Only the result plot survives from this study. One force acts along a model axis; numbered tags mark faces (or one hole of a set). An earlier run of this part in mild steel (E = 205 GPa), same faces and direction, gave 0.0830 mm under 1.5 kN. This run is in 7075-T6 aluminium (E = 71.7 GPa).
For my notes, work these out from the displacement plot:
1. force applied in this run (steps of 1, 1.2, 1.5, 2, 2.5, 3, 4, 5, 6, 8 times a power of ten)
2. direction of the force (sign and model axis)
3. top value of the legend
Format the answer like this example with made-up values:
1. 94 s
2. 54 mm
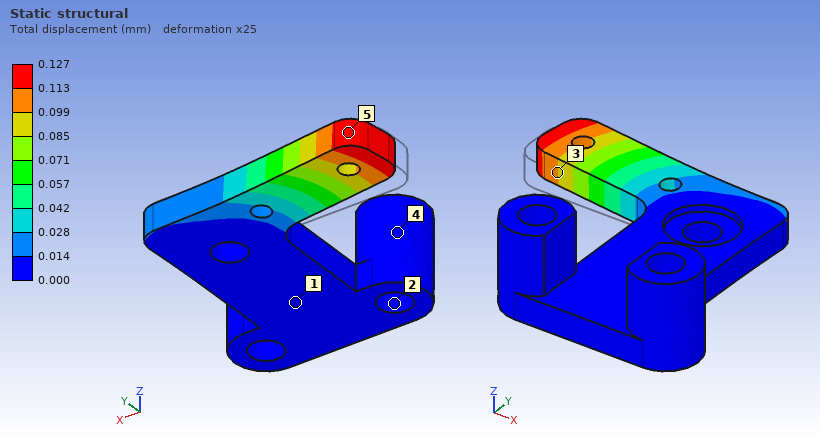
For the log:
1. 800 N
2. +Y
3. 0.127 mm
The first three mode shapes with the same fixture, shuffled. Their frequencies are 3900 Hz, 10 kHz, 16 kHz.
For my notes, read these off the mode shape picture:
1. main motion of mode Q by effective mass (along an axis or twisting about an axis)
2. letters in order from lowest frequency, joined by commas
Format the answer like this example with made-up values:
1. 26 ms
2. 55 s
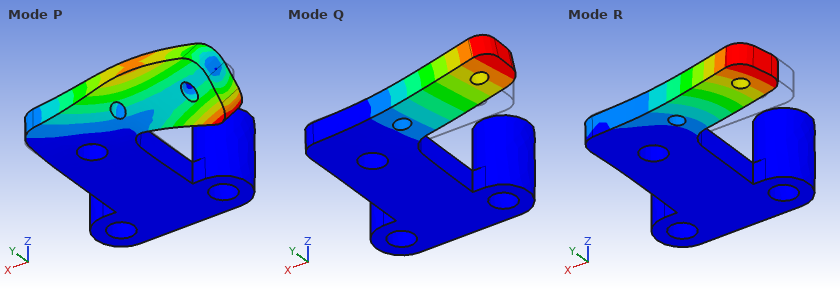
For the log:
1. along Z
2. Q, R, P
